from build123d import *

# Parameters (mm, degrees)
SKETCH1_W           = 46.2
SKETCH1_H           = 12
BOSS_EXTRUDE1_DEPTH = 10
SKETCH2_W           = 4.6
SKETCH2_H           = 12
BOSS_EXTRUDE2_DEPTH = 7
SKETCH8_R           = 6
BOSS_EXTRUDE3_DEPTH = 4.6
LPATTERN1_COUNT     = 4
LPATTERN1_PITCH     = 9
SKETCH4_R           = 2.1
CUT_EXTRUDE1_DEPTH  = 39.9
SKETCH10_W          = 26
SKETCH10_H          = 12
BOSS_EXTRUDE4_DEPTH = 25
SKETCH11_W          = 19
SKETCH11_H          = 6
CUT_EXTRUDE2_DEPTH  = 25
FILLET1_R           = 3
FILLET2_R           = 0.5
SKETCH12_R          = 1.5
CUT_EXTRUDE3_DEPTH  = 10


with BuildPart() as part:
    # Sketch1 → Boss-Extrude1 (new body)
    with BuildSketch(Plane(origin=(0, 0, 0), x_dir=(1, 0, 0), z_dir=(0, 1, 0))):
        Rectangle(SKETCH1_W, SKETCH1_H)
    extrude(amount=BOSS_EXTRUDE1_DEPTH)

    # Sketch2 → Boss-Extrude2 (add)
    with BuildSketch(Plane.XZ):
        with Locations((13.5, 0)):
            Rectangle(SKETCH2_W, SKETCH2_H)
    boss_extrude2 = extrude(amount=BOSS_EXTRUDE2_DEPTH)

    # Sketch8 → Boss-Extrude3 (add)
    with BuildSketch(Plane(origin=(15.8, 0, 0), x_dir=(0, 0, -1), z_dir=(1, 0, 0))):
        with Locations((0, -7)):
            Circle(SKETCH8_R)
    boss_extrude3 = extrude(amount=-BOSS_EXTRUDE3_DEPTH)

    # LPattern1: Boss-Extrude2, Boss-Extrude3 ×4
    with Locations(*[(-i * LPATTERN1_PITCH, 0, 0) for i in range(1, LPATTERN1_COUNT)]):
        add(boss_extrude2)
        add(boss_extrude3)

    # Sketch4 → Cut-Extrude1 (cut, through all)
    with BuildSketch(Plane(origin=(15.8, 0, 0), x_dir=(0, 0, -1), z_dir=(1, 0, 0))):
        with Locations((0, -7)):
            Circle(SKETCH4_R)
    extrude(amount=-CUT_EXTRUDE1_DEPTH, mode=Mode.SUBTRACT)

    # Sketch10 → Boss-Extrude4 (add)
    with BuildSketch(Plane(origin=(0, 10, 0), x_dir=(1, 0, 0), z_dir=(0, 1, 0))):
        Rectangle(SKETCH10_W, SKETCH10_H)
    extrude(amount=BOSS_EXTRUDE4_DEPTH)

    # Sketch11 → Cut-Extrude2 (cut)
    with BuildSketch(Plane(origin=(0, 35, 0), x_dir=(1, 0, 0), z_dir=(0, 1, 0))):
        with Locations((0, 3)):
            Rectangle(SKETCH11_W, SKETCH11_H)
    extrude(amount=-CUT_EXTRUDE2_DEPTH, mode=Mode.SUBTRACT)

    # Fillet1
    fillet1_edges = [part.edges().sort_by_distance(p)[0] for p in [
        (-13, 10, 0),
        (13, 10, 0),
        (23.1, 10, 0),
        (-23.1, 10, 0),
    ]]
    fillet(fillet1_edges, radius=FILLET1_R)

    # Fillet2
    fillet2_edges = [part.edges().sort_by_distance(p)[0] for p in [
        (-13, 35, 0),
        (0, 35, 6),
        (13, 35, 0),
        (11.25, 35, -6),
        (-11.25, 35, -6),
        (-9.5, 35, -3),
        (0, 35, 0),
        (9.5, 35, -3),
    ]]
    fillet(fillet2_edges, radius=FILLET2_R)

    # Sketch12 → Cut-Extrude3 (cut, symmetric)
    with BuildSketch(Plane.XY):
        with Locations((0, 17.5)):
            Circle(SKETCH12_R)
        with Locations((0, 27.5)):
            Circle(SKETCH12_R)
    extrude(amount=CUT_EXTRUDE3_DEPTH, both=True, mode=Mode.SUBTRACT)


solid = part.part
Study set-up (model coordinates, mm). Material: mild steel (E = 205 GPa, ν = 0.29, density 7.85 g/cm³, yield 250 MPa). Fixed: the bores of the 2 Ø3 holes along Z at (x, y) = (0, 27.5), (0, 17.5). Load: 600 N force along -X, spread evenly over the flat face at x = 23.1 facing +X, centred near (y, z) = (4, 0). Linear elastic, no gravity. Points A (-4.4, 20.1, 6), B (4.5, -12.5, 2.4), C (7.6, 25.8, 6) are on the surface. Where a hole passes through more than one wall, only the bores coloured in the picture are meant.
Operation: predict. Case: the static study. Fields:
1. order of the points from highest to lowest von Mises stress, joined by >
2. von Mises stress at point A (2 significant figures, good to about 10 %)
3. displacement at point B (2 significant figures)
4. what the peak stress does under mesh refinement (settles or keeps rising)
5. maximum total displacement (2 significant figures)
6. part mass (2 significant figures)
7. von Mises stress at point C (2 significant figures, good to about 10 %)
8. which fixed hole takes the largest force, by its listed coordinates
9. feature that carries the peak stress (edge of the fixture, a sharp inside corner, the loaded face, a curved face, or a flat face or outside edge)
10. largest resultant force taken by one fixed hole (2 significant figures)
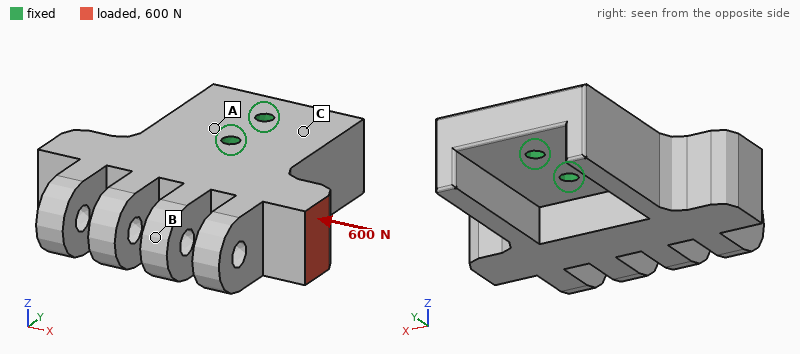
A > C > B
12 MPa
4.4 µm
keeps rising
6.4 µm
100 g
8.6 MPa
(0, 17.5)
edge of the fixture
1.2 kN
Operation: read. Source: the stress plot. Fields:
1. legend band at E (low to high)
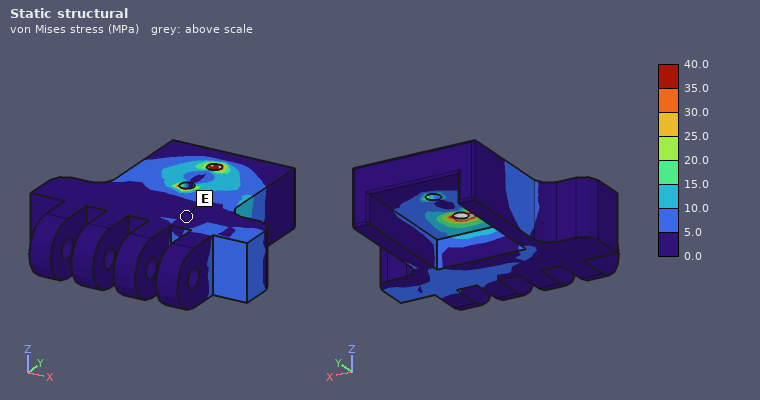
0.0 to 5.0 MPa
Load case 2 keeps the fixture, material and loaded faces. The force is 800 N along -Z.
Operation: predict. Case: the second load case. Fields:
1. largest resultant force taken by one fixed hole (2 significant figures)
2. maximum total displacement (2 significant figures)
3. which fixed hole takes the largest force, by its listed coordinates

1.3 kN
49 µm
(0, 17.5)
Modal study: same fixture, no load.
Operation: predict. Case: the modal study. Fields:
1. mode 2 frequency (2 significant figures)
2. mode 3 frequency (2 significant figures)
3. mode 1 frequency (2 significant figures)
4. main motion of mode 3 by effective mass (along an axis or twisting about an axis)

5400 Hz
7300 Hz
5300 Hz
along X
